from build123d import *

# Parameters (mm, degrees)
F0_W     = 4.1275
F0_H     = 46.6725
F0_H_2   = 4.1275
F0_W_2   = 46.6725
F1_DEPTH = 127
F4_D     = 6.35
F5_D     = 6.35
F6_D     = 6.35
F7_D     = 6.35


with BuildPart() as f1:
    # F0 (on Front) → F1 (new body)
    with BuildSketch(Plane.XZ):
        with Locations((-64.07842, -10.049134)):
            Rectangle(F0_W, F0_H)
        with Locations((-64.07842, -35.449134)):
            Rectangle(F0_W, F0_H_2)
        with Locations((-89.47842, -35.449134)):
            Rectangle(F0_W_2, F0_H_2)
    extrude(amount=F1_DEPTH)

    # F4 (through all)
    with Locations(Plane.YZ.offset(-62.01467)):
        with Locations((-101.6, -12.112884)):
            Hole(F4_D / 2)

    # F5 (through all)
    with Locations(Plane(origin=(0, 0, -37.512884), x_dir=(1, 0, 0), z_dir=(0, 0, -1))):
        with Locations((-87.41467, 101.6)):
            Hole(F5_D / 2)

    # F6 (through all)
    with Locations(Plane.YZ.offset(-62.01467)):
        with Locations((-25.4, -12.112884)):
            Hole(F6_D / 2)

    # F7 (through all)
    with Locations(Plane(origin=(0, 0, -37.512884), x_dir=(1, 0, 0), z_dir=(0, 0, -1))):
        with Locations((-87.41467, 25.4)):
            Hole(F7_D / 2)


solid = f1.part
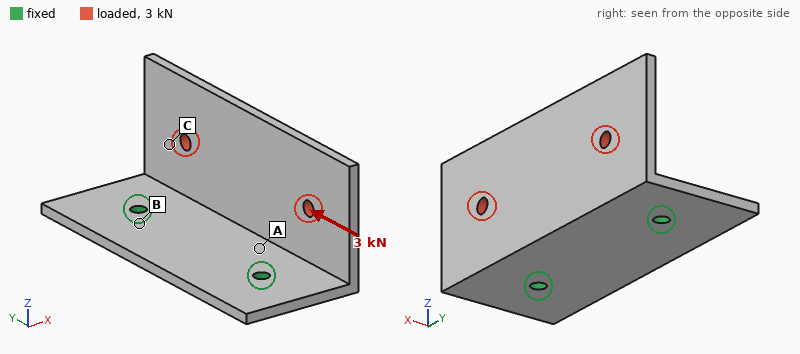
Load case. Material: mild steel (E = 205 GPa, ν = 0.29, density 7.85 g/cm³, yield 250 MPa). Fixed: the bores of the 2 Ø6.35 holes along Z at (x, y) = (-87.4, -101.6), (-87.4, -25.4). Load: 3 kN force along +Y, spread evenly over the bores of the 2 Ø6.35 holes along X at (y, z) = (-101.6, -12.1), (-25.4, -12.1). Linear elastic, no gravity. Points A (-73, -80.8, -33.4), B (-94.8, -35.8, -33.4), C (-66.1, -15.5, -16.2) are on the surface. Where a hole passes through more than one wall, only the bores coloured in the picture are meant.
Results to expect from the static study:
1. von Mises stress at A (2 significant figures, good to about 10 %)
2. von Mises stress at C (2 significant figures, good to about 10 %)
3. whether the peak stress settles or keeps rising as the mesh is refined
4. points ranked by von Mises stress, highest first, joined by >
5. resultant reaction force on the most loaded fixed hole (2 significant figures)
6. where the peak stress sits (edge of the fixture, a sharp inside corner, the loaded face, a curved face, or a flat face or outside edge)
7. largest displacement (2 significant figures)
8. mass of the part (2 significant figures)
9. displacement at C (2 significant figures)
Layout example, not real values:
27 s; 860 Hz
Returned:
49 MPa; 28 MPa; keeps rising; A > C > B; 1.9 kN; edge of the fixture; 0.13 mm; 400 g; 0.069 mm
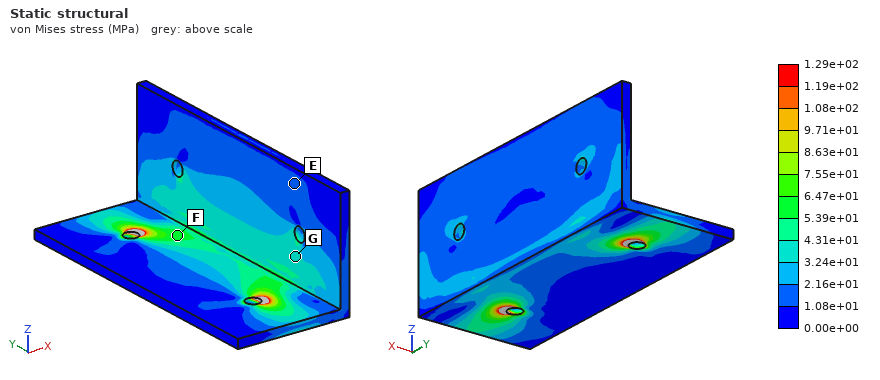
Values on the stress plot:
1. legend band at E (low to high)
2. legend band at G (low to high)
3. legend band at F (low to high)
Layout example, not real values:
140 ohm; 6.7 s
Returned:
1.08e+01 to 2.16e+01 MPa; 3.24e+01 to 4.31e+01 MPa; 5.39e+01 to 6.47e+01 MPa
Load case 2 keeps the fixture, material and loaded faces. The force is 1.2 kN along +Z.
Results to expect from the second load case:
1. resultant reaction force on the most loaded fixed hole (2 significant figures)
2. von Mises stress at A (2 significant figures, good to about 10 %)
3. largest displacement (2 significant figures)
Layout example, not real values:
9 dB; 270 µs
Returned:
600 N; 26 MPa; 0.14 mm
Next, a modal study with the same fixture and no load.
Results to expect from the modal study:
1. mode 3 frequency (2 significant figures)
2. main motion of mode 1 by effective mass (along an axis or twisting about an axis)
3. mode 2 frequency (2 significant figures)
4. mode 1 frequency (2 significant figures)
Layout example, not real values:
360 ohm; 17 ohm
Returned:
2300 Hz; along X; 1300 Hz; 770 Hz
